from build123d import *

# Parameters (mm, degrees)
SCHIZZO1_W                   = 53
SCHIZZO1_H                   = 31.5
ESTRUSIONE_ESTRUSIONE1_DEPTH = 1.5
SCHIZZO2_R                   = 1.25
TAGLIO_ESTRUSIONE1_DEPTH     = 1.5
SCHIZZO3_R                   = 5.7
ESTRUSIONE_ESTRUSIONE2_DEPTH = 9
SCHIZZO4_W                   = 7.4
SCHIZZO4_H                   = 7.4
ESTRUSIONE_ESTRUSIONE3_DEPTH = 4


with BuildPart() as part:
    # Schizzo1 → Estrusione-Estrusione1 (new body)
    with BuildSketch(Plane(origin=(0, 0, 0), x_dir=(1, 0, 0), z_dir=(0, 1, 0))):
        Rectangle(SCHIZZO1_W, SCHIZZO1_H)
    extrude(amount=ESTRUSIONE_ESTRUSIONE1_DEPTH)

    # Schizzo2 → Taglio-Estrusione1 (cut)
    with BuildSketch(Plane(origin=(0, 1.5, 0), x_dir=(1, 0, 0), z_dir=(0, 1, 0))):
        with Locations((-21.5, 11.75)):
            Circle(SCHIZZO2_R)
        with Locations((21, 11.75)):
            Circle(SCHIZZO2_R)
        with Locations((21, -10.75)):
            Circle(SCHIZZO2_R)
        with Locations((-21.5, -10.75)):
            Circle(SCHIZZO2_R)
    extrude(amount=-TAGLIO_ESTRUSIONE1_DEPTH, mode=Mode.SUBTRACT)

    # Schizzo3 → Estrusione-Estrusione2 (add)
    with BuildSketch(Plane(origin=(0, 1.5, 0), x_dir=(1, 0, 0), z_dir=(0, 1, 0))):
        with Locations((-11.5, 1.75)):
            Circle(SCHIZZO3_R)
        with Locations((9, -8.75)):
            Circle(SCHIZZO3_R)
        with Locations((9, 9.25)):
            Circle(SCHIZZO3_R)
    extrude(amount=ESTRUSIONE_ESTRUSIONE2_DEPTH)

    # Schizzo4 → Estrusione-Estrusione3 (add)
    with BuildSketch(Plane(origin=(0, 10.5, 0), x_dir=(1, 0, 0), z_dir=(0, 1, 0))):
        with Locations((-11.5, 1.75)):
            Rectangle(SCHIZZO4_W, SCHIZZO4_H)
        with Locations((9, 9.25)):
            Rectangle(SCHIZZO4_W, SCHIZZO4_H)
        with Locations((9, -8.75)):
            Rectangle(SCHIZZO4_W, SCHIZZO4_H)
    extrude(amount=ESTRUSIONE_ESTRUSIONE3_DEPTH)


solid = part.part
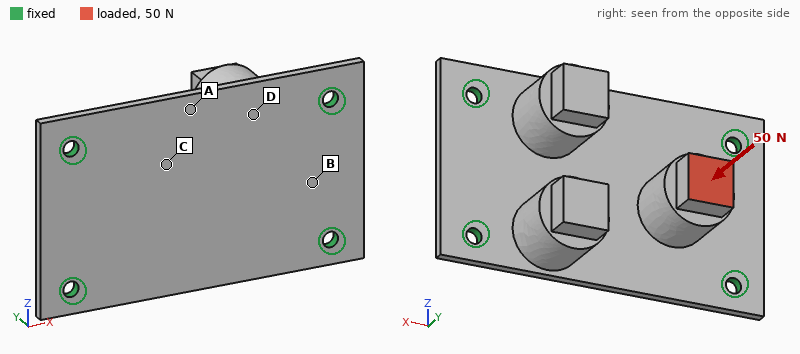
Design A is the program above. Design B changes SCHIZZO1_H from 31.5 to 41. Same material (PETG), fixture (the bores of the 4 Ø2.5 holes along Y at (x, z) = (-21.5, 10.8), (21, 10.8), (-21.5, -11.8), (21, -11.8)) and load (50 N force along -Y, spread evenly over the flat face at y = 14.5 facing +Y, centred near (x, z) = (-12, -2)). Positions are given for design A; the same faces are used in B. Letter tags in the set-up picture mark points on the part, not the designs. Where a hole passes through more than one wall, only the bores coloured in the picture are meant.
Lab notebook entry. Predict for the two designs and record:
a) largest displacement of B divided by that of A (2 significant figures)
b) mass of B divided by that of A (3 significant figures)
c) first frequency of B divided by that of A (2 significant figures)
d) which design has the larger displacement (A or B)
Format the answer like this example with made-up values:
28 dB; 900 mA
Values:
0.89; 1.13; 1.1; A
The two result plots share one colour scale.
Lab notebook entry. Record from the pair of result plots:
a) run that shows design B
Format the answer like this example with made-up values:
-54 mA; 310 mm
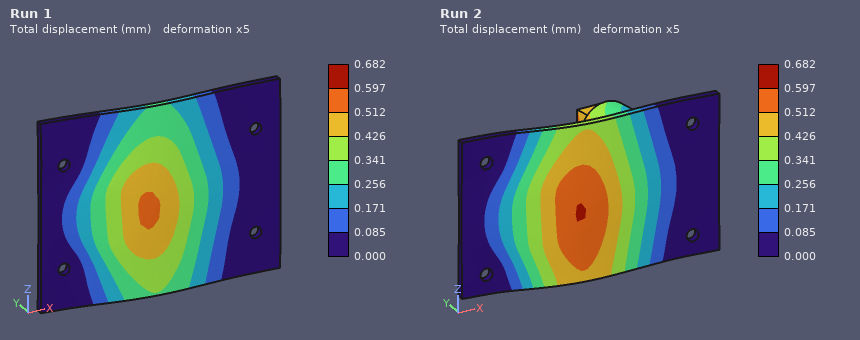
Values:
Run 1
